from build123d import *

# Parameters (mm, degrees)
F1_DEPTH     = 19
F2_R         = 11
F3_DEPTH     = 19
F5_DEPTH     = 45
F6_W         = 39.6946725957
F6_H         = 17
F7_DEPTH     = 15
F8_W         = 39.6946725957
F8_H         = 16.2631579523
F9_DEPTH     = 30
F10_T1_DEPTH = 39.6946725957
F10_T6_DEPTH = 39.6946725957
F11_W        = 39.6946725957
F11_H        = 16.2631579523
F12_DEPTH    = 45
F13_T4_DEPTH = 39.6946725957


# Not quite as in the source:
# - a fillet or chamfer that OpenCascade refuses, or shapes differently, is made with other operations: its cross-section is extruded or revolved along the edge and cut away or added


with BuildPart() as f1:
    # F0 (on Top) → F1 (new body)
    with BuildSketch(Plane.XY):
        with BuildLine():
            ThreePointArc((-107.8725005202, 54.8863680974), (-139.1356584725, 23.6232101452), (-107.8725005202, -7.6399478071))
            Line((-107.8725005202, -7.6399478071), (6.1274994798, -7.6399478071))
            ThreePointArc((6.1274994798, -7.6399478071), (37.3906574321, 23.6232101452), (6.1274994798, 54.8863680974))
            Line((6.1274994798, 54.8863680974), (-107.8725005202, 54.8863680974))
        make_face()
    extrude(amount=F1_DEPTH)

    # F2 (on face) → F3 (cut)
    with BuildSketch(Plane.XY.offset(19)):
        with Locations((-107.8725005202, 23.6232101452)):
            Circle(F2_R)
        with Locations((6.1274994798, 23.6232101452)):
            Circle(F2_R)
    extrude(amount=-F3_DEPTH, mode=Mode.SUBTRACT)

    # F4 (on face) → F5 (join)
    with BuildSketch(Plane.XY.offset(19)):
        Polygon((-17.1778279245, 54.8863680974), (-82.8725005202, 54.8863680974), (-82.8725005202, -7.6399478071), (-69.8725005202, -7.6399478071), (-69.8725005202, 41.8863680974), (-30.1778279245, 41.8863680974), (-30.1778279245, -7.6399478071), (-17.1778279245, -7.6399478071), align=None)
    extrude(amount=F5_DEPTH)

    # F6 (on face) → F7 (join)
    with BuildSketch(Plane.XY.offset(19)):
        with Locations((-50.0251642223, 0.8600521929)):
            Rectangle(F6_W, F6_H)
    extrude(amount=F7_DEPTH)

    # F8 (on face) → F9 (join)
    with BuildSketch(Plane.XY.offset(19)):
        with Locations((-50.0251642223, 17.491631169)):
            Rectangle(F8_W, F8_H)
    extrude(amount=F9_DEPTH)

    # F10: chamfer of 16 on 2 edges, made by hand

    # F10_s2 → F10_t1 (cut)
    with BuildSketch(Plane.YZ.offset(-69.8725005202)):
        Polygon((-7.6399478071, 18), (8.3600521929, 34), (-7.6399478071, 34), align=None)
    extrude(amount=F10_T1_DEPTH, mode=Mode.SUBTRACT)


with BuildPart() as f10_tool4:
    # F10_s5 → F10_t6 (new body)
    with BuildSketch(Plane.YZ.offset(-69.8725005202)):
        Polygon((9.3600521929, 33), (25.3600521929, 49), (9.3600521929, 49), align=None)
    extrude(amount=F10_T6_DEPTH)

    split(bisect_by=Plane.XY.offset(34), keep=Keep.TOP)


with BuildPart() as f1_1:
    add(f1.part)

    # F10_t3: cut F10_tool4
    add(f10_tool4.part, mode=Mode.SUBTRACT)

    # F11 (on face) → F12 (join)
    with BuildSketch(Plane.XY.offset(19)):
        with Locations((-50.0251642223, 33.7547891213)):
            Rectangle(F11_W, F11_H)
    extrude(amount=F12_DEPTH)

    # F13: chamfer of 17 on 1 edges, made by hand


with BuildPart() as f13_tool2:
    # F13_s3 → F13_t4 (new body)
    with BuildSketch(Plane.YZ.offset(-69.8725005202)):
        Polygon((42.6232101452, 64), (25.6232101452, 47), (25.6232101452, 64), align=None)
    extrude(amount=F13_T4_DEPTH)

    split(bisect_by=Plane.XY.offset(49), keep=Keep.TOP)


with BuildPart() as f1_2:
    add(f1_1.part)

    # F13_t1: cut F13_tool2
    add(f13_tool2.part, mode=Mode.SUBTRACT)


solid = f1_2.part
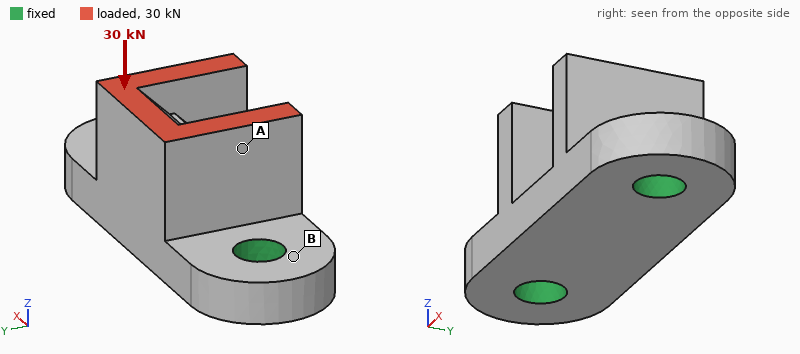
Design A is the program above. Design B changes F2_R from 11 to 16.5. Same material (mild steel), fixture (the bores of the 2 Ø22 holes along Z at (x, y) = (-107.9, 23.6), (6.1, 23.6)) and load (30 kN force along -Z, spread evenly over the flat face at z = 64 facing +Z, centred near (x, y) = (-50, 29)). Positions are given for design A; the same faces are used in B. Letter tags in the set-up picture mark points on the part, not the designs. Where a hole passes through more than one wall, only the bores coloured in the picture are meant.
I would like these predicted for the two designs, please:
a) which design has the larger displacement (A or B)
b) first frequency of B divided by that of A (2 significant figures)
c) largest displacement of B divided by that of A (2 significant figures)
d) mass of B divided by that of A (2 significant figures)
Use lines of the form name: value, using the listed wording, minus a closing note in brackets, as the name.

which design has the larger displacement: A
first frequency of B divided by that of A: 1.2
largest displacement of B divided by that of A: 0.70
mass of B divided by that of A: 0.94
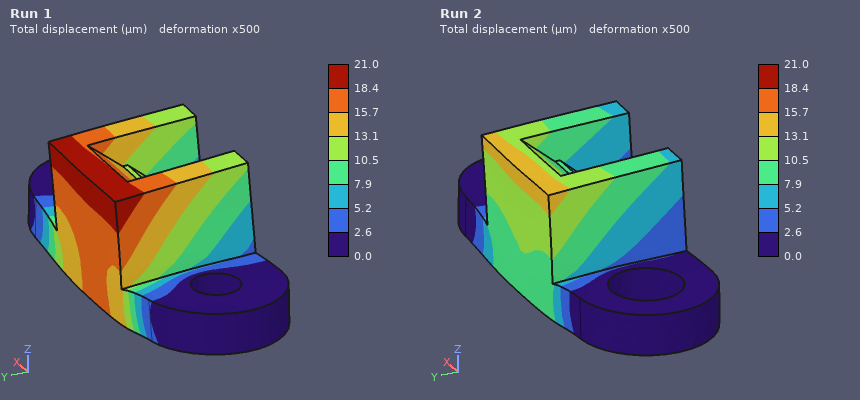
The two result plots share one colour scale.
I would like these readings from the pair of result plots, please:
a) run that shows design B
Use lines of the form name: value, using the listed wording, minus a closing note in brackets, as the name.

run that shows design B: Run 2
